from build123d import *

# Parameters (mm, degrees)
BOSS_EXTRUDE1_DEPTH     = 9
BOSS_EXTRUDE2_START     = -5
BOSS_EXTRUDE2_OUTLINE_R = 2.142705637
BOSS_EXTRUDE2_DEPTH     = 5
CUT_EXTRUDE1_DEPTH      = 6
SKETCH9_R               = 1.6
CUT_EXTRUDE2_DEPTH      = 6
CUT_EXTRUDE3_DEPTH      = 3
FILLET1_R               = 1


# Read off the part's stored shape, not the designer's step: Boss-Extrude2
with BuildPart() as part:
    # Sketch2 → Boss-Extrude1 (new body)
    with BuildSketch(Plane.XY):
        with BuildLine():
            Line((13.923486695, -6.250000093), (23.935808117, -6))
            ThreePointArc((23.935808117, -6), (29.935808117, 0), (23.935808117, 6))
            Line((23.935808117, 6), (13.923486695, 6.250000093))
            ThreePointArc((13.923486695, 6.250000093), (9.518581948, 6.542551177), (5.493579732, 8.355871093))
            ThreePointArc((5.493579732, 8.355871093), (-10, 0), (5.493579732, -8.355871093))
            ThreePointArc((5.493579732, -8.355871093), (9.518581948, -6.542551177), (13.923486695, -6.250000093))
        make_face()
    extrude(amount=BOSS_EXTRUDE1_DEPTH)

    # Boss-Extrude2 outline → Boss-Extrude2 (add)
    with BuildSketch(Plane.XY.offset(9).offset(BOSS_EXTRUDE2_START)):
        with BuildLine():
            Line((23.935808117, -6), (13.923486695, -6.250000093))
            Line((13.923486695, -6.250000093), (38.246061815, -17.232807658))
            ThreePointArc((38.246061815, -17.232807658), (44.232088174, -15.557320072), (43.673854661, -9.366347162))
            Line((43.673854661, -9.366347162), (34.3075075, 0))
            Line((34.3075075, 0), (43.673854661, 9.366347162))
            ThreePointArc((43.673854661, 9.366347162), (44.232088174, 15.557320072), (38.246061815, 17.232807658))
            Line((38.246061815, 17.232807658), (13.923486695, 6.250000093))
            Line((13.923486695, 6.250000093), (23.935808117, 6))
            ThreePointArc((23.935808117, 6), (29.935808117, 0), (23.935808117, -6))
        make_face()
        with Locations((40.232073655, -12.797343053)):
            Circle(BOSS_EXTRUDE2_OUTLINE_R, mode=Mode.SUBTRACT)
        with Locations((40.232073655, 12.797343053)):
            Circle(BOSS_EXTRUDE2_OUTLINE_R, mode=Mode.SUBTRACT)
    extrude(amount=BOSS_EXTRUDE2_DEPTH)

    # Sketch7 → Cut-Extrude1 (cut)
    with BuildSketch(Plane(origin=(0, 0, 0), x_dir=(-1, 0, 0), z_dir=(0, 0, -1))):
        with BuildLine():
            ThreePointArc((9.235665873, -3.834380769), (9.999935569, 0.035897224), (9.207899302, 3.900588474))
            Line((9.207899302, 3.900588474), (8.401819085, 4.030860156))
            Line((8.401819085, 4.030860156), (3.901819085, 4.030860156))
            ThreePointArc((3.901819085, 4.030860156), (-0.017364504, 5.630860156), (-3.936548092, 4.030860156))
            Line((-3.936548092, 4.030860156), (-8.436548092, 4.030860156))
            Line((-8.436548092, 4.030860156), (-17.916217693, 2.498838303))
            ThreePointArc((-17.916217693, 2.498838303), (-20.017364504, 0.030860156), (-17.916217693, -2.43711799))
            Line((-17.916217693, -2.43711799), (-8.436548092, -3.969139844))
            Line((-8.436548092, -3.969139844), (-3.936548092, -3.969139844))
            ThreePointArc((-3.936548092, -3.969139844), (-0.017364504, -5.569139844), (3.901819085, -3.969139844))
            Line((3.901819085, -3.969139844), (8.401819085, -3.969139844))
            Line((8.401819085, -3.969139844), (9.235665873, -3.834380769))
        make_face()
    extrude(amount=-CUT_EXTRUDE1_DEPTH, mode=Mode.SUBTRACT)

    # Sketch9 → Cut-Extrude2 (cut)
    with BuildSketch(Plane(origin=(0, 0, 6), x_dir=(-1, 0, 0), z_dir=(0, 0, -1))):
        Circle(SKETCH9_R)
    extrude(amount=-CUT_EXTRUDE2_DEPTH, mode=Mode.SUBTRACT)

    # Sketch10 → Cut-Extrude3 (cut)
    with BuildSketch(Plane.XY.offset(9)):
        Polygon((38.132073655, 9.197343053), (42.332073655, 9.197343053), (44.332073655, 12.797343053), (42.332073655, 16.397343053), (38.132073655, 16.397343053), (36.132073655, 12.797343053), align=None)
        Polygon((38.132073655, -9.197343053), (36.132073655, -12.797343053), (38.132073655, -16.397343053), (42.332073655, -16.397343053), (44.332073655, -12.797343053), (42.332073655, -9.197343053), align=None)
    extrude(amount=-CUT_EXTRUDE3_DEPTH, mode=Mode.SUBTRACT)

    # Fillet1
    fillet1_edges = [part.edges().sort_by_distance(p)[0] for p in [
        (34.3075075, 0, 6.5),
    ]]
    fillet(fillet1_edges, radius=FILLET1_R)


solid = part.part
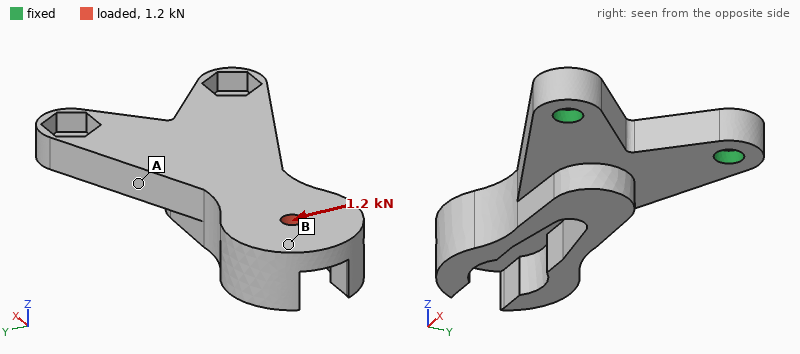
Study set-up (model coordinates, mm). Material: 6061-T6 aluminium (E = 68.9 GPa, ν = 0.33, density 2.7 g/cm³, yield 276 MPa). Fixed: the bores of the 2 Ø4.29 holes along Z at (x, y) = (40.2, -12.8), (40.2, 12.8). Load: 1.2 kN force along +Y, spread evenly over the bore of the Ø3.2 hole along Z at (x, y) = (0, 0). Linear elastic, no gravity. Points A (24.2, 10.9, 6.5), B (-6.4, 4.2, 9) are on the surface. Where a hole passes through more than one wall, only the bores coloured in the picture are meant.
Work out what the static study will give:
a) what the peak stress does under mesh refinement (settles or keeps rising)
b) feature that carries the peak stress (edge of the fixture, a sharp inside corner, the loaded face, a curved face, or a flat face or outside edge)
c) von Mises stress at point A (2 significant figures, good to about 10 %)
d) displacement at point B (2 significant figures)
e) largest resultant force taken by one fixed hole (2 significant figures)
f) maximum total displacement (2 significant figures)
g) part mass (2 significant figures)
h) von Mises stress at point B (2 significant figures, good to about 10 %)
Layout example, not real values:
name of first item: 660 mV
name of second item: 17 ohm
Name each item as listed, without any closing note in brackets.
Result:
what the peak stress does under mesh refinement: keeps rising
feature that carries the peak stress: edge of the fixture
von Mises stress at point A: 77 MPa
displacement at point B: 0.15 mm
largest resultant force taken by one fixed hole: 1.9 kN
maximum total displacement: 0.19 mm
part mass: 16 g
von Mises stress at point B: 28 MPa
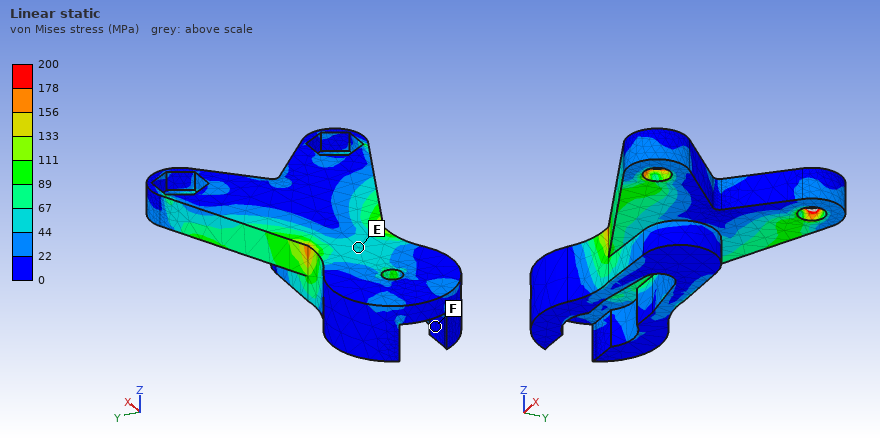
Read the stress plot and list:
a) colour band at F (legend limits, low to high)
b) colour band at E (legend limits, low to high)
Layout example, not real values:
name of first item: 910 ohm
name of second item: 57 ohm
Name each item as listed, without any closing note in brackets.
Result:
colour band at F: 0 to 22 MPa
colour band at E: 44 to 67 MPa
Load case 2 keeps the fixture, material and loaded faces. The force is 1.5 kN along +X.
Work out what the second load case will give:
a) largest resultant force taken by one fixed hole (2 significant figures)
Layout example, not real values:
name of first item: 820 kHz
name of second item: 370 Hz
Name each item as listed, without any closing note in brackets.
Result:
largest resultant force taken by one fixed hole: 810 N
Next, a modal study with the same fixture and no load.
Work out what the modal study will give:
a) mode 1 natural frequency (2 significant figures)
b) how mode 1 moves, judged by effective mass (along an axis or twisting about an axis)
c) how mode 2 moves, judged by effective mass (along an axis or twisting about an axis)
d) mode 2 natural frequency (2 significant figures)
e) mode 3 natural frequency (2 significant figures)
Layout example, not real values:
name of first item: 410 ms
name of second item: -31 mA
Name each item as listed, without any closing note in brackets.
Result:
mode 1 natural frequency: 1400 Hz
how mode 1 moves, judged by effective mass: along Z
how mode 2 moves, judged by effective mass: along Y
mode 2 natural frequency: 5700 Hz
mode 3 natural frequency: 9100 Hz
